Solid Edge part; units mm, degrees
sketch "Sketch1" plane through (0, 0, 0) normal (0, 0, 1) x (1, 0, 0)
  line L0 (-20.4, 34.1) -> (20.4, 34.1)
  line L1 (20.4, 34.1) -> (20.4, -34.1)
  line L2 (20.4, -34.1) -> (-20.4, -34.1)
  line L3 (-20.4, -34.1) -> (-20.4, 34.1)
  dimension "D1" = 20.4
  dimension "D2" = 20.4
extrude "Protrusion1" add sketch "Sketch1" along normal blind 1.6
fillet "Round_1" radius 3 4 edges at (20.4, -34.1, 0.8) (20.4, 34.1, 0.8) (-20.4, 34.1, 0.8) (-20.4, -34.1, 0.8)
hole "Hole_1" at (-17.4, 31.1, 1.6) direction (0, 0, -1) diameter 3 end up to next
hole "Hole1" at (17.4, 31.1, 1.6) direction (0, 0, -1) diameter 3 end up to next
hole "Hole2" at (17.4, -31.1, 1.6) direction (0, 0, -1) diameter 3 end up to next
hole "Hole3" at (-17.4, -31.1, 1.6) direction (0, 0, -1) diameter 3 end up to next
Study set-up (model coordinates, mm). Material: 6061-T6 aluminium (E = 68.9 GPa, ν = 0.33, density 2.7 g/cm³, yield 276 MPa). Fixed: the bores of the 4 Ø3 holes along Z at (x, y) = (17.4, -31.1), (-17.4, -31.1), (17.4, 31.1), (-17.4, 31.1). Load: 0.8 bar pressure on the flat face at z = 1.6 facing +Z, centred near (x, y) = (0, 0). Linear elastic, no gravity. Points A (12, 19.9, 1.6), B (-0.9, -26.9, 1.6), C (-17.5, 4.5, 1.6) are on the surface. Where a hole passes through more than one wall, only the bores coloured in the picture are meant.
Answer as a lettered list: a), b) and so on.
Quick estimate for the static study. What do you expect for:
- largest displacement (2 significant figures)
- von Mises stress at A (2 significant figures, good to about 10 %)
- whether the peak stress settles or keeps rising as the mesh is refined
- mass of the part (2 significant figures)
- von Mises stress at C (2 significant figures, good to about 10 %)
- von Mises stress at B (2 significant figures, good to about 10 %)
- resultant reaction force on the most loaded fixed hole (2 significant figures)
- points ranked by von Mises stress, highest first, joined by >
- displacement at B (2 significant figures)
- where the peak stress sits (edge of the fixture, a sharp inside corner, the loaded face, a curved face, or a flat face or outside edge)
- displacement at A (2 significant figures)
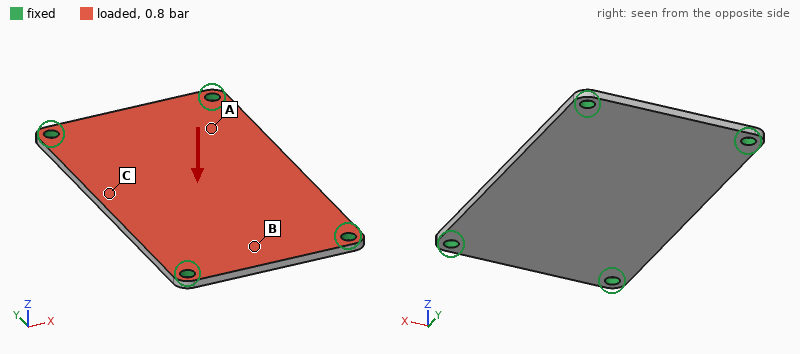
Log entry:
a) 0.17 mm
b) 9.5 MPa
c) keeps rising
d) 12 g
e) 34 MPa
f) 17 MPa
g) 55 N
h) C > B > A
i) 0.039 mm
j) edge of the fixture
k) 0.070 mm
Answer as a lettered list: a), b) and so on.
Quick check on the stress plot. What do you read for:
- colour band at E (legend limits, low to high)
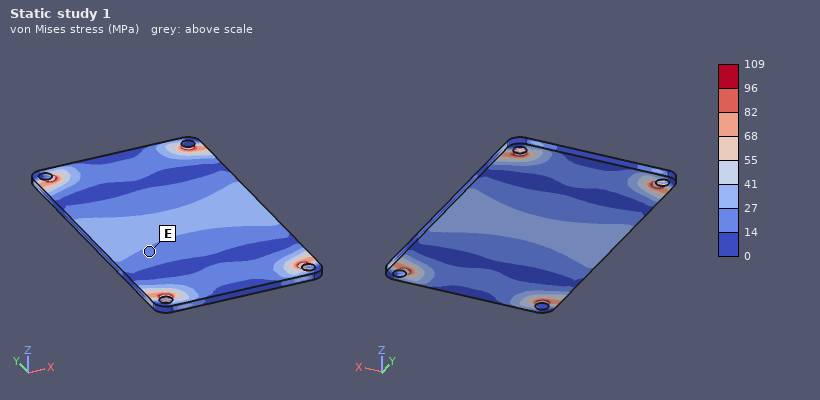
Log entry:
a) 14 to 27 MPa
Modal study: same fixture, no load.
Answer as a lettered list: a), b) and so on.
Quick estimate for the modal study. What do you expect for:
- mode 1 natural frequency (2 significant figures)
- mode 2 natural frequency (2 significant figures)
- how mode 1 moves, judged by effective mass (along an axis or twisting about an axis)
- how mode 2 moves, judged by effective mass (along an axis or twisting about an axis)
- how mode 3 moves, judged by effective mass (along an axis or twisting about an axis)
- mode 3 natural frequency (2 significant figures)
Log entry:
a) 1900 Hz
b) 3100 Hz
c) along Z
d) twisting about Y
e) twisting about X
f) 5100 Hz
